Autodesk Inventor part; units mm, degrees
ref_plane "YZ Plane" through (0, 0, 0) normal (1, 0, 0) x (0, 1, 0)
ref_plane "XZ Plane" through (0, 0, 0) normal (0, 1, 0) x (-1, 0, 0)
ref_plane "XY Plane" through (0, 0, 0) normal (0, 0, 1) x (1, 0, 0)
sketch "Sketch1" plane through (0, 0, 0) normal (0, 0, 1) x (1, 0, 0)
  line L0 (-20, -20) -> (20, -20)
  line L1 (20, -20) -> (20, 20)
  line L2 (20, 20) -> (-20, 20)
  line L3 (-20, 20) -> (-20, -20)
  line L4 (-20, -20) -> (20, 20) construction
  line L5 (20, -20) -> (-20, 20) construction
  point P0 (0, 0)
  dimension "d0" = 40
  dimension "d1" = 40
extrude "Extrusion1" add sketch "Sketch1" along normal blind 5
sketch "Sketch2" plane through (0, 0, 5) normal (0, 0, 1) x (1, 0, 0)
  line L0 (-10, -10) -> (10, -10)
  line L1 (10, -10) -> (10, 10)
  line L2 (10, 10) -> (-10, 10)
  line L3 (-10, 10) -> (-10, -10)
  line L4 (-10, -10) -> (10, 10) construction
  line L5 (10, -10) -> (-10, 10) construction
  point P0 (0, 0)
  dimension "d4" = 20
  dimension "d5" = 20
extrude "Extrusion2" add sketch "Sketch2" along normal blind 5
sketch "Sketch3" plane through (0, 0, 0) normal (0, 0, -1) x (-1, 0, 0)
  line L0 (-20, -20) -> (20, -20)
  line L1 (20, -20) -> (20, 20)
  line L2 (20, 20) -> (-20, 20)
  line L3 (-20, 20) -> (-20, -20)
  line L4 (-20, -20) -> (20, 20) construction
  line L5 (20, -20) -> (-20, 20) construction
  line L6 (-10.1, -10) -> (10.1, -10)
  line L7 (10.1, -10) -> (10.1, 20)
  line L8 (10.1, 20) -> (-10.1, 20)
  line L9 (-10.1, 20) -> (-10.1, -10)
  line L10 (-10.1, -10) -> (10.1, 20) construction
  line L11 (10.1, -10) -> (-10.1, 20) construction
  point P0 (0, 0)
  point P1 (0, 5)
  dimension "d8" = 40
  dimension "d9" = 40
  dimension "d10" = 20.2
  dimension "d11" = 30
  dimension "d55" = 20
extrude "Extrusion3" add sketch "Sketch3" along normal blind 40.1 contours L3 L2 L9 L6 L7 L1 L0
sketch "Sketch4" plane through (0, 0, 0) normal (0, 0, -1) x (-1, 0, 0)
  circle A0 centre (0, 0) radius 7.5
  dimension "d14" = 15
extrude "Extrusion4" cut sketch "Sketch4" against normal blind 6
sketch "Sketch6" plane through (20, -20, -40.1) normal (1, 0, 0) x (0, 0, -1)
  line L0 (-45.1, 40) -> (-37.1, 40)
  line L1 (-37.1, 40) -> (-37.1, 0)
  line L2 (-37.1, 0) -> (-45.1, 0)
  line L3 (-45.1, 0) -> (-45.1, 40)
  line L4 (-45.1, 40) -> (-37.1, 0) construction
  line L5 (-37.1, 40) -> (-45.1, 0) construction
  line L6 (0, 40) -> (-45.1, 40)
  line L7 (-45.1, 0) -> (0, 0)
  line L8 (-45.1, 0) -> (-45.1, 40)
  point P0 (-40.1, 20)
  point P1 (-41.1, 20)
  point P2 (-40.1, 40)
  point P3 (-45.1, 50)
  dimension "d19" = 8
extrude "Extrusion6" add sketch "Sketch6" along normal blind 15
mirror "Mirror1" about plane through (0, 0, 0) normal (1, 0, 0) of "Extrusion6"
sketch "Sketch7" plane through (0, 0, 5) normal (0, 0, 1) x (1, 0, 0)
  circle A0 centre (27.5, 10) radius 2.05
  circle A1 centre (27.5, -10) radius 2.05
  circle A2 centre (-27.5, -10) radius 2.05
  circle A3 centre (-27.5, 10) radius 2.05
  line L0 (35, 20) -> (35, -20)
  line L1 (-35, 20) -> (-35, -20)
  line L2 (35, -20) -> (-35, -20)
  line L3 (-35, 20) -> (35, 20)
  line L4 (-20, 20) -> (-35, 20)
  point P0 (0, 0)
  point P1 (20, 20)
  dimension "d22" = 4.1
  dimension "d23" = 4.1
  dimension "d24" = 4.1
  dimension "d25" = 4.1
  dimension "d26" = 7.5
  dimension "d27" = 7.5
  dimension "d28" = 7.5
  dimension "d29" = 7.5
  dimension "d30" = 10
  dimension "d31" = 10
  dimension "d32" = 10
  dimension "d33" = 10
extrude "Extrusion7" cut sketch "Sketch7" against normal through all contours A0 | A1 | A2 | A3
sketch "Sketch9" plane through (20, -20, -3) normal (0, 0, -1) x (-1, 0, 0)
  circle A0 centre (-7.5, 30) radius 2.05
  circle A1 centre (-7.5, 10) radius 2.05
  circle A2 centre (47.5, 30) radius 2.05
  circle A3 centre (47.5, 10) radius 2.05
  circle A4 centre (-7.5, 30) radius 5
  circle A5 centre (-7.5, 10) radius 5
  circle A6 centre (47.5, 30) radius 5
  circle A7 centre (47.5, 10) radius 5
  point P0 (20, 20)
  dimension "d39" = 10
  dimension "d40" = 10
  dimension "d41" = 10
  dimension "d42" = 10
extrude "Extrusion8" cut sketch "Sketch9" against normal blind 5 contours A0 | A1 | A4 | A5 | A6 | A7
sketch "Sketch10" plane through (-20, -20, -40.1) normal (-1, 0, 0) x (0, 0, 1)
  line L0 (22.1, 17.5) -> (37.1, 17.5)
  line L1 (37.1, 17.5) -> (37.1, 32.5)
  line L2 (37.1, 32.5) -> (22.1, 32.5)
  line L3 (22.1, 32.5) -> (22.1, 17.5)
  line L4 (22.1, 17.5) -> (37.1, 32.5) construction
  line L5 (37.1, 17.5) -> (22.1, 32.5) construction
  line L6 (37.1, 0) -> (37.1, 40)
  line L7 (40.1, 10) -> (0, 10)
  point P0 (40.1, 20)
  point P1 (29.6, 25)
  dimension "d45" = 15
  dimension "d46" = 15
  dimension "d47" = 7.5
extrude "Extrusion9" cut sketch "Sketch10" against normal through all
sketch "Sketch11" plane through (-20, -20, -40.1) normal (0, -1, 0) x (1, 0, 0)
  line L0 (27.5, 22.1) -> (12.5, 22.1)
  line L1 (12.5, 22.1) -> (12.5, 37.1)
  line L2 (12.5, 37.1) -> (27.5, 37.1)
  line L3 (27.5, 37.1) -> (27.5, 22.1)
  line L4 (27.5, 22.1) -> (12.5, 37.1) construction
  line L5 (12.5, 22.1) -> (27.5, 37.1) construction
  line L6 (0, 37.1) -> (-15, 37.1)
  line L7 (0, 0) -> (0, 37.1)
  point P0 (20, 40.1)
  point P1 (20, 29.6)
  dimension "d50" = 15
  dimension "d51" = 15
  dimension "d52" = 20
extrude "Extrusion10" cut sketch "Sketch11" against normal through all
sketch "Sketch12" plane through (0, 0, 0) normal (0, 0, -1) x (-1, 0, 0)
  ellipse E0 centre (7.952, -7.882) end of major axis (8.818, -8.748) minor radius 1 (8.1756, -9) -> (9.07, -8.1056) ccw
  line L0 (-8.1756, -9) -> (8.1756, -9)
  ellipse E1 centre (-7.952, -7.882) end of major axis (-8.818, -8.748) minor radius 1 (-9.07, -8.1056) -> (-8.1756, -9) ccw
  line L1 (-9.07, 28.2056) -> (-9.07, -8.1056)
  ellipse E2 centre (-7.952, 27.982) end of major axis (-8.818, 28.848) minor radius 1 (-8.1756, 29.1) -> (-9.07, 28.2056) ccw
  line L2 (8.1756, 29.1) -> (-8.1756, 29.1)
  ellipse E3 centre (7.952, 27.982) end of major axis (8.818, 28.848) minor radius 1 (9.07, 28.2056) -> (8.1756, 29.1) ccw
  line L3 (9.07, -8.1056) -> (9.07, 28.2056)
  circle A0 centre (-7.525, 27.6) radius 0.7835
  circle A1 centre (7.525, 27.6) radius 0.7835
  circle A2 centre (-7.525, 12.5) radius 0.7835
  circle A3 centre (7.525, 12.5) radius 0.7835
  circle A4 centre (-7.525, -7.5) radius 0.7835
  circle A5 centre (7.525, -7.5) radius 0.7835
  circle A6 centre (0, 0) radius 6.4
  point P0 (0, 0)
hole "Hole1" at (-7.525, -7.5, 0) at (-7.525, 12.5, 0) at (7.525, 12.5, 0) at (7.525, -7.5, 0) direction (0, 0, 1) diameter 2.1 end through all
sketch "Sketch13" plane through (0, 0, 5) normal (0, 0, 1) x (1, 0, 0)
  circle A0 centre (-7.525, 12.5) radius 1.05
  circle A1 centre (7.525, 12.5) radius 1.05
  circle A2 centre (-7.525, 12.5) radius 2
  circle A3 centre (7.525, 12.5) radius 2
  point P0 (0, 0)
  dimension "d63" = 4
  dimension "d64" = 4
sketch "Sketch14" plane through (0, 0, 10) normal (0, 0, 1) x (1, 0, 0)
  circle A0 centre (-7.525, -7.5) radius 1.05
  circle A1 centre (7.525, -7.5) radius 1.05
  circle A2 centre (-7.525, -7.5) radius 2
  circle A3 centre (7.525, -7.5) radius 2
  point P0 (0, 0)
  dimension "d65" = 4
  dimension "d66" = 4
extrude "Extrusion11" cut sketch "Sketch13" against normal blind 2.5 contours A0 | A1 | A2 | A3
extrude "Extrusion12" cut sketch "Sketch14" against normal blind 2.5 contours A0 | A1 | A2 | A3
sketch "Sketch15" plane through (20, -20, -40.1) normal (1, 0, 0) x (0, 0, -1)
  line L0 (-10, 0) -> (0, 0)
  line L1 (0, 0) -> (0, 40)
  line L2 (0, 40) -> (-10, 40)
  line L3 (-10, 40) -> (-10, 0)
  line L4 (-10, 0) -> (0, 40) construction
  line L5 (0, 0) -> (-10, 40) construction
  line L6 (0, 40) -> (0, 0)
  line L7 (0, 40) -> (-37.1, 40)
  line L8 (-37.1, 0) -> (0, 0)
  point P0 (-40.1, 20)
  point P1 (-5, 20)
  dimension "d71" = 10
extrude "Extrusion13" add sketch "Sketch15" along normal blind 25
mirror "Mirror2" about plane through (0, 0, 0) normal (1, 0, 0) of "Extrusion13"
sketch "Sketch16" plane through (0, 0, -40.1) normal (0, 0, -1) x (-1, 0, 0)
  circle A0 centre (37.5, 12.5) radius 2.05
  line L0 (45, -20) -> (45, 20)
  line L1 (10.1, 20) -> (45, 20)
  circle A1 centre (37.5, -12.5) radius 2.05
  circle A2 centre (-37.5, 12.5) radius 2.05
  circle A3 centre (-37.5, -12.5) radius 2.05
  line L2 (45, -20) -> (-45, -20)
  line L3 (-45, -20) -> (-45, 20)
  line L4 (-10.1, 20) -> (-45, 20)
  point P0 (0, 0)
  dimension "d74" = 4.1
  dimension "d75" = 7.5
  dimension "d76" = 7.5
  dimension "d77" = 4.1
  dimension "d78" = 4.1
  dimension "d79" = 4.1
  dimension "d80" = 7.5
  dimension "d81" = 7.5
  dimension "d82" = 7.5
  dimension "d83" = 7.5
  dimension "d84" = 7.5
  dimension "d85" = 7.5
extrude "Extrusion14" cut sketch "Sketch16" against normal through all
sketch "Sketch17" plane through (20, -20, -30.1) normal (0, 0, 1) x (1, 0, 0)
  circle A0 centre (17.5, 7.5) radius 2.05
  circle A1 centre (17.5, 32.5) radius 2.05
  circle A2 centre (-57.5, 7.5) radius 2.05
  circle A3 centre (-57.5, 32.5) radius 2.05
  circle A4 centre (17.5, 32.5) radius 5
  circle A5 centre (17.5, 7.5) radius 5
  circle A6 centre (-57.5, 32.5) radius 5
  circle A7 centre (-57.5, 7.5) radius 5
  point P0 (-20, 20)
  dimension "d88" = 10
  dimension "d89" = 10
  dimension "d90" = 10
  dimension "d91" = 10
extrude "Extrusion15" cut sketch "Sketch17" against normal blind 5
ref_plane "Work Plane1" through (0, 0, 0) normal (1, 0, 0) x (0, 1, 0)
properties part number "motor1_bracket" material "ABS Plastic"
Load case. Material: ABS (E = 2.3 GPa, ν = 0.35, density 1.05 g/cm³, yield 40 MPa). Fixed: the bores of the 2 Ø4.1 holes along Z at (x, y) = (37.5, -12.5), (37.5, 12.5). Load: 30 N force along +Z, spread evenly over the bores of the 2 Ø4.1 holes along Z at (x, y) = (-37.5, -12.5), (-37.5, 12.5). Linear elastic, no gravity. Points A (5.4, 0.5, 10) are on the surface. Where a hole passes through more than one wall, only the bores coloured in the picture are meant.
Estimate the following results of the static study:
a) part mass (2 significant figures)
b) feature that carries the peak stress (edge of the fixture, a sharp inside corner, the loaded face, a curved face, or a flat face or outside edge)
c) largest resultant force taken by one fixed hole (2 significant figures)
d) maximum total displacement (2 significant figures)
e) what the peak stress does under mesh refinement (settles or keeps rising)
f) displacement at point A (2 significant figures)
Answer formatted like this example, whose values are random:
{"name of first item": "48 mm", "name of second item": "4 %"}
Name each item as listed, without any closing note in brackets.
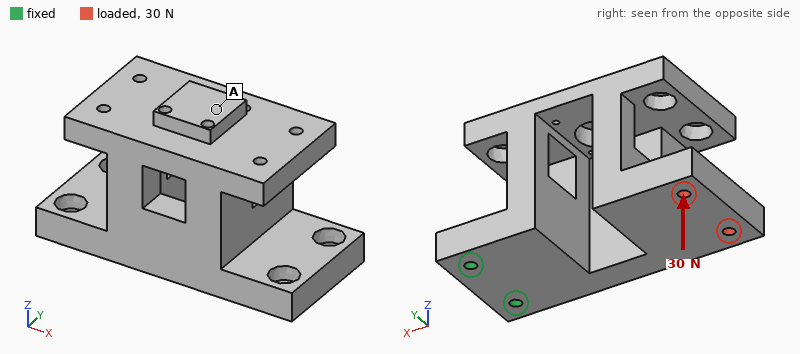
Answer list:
{"part mass": "71 g", "feature that carries the peak stress": "edge of the fixture", "largest resultant force taken by one fixed hole": "16 N", "maximum total displacement": "1.0 mm", "what the peak stress does under mesh refinement": "keeps rising", "displacement at point A": "0.67 mm"}
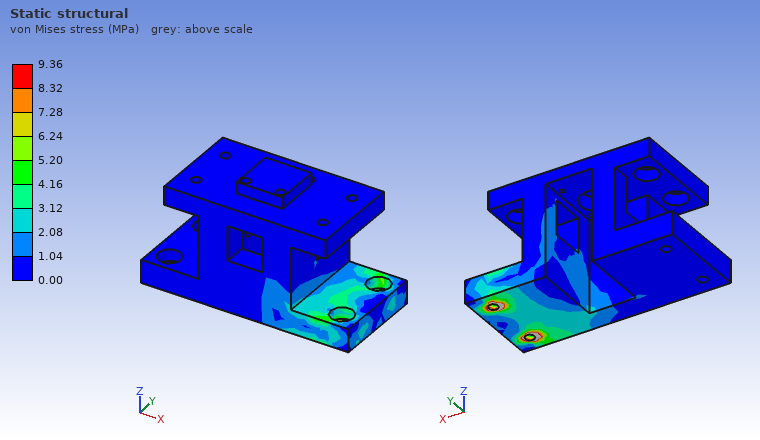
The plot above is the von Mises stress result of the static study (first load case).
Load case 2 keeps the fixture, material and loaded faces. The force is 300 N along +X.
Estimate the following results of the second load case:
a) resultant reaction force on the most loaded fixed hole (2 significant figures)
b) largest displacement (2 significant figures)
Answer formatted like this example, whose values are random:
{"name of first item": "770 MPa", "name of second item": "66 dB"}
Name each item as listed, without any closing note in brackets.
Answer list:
{"resultant reaction force on the most loaded fixed hole": "150 N", "largest displacement": "1.3 mm"}
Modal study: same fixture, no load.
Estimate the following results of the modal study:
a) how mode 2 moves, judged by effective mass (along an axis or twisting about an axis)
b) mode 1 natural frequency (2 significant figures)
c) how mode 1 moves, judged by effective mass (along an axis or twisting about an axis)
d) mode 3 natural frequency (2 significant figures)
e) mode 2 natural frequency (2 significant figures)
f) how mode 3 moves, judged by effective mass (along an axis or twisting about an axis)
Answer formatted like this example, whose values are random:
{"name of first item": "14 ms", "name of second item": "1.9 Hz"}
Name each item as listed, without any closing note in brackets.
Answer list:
{"how mode 2 moves, judged by effective mass": "along Y", "mode 1 natural frequency": "170 Hz", "how mode 1 moves, judged by effective mass": "along Z", "mode 3 natural frequency": "600 Hz", "mode 2 natural frequency": "420 Hz", "how mode 3 moves, judged by effective mass": "along Y"}
